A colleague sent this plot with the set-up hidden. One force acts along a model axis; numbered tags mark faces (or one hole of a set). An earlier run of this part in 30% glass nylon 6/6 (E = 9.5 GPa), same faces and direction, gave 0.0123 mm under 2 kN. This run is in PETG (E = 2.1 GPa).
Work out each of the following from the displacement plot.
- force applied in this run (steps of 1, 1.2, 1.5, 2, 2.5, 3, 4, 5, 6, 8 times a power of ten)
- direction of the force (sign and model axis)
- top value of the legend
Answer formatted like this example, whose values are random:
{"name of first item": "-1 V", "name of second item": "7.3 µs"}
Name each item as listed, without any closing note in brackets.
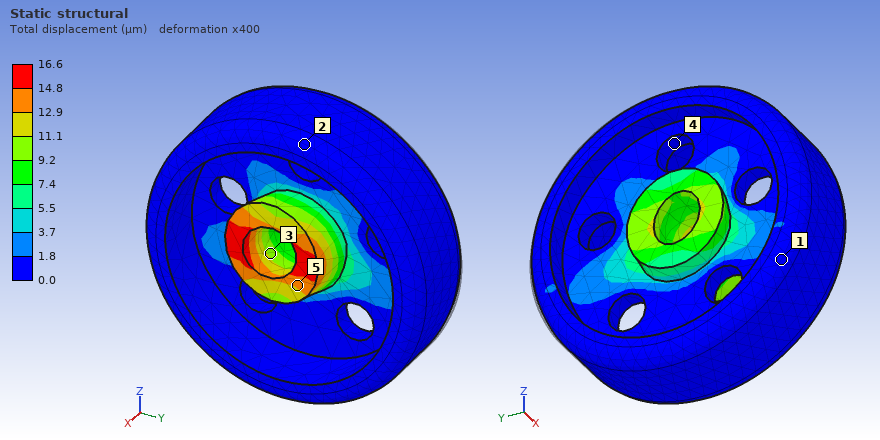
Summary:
{"force applied in this run": "600 N", "direction of the force": "-Y", "top value of the legend": "16.6 µm"}
